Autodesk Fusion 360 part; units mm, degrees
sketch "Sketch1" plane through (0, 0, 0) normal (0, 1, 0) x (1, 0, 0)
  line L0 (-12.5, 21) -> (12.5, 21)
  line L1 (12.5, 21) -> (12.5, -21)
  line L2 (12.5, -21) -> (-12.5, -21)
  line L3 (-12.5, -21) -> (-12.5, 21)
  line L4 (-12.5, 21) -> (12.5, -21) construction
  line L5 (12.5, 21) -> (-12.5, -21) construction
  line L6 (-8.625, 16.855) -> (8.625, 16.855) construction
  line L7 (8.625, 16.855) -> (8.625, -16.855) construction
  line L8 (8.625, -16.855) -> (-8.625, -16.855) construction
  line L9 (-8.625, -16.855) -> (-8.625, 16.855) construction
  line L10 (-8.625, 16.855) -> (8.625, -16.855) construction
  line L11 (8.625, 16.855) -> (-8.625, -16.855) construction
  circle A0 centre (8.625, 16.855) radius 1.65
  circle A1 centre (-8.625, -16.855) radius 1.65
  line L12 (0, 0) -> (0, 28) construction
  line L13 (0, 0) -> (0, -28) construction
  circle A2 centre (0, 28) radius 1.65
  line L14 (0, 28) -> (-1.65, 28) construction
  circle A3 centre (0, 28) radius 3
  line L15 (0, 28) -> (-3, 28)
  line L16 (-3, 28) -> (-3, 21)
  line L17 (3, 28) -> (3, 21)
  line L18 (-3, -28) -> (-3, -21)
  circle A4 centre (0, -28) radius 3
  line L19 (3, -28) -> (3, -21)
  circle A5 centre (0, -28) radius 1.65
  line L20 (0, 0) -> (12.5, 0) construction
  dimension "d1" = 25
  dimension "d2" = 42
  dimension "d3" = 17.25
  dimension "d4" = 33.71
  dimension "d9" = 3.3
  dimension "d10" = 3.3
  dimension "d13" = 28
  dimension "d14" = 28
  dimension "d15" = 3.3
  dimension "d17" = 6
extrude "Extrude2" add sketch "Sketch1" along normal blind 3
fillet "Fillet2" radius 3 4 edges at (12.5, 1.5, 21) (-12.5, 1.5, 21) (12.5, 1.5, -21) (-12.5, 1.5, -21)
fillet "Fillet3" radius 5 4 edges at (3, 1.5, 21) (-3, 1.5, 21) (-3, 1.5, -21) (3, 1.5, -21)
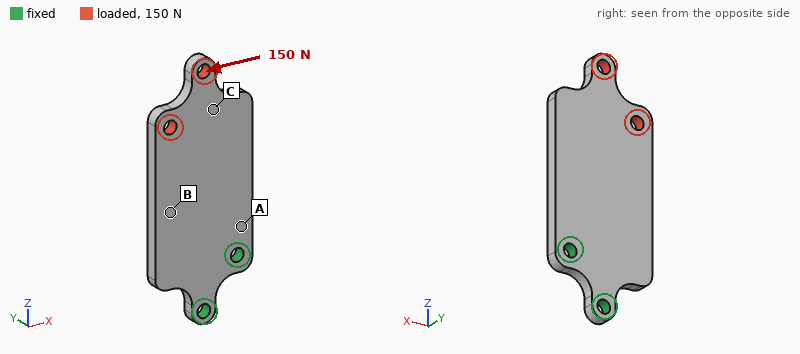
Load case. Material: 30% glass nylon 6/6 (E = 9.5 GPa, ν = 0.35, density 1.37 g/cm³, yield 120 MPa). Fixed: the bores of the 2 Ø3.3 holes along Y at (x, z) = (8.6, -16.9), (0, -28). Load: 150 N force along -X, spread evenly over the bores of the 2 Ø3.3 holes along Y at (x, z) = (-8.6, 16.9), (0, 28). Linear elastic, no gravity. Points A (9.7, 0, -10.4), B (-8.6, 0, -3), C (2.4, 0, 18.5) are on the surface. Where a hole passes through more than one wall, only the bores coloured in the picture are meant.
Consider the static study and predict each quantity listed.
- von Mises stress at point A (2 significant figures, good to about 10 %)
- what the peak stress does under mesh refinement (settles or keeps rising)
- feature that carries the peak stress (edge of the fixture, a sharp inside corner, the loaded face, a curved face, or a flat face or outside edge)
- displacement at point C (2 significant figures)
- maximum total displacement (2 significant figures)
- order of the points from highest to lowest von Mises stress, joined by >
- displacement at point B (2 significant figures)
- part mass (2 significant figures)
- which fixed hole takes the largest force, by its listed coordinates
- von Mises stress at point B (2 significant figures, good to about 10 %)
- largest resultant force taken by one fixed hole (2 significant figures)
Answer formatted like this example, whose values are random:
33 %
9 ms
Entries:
17 MPa
keeps rising
edge of the fixture
0.21 mm
0.33 mm
A > B > C
0.099 mm
4.7 g
(8.6, -16.9)
8.3 MPa
500 N
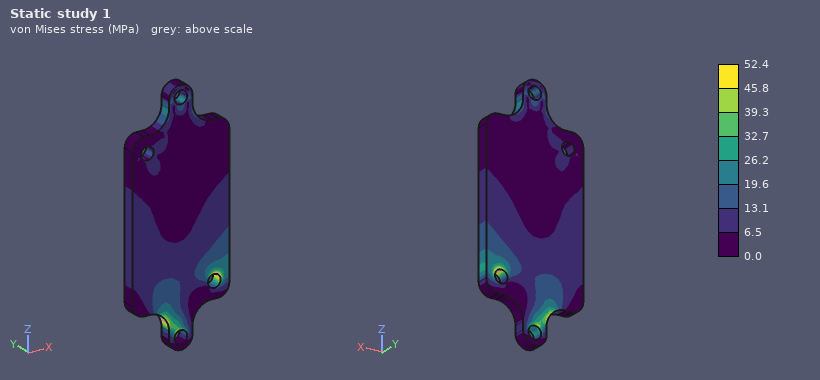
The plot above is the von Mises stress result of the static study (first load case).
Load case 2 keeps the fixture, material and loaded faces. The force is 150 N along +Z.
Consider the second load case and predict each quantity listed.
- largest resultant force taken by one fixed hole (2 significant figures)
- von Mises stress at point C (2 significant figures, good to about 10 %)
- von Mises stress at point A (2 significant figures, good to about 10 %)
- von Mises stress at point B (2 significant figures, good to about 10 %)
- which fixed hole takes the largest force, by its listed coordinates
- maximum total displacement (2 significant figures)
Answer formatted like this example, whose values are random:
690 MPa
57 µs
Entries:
150 N
2.3 MPa
1.4 MPa
3.4 MPa
(0, -28)
69 µm
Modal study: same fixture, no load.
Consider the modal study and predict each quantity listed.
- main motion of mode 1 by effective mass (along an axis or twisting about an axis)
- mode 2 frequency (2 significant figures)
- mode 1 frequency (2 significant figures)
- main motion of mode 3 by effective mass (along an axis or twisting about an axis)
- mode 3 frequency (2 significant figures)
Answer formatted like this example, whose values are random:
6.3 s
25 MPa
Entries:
along Y
2100 Hz
690 Hz
along X
3300 Hz
